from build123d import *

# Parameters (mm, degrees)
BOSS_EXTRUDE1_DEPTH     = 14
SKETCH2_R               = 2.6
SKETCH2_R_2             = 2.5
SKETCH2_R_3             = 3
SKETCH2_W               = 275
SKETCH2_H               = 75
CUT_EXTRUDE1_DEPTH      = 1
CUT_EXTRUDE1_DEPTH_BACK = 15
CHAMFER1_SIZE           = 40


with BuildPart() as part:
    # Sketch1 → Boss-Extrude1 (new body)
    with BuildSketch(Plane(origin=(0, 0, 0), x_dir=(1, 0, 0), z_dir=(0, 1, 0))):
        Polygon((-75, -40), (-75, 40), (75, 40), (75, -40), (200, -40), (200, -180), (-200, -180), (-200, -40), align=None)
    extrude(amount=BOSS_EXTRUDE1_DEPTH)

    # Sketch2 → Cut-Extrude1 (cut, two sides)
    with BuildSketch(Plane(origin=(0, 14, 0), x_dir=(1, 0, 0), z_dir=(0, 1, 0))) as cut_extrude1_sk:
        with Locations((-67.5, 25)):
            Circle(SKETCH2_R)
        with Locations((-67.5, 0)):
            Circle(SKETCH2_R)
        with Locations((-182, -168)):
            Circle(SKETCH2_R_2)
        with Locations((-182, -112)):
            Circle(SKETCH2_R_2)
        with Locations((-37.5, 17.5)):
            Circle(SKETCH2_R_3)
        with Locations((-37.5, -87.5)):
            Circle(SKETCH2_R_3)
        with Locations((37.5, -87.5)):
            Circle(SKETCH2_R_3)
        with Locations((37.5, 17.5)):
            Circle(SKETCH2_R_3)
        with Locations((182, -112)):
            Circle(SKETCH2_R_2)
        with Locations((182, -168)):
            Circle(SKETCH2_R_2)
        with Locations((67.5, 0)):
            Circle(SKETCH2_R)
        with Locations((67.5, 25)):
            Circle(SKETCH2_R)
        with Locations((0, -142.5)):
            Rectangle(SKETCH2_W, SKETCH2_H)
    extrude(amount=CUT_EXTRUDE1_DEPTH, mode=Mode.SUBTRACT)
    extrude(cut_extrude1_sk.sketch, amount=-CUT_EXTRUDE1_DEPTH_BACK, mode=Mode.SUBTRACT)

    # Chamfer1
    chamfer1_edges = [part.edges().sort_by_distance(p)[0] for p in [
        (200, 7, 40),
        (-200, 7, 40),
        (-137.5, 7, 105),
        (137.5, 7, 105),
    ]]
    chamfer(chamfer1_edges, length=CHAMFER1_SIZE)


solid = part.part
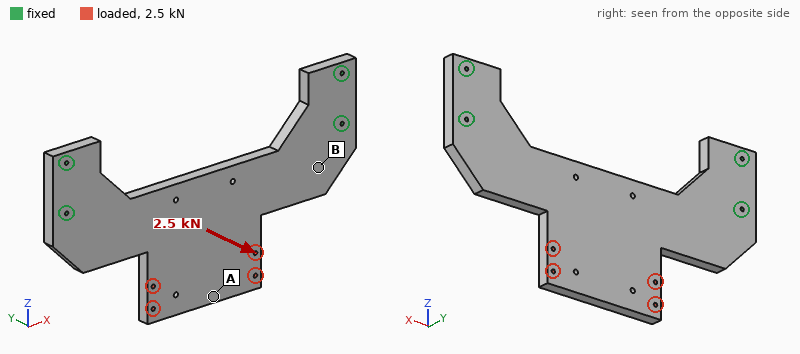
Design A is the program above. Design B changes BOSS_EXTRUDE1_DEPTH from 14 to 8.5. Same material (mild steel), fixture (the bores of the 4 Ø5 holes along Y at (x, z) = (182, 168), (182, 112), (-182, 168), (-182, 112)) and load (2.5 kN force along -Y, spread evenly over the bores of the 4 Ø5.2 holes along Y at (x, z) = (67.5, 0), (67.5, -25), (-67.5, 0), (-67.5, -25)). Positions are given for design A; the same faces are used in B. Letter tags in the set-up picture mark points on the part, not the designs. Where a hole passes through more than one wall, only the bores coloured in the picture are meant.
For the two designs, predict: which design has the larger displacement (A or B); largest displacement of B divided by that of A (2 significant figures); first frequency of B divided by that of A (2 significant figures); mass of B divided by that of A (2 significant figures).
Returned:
B
4.2
0.63
0.61
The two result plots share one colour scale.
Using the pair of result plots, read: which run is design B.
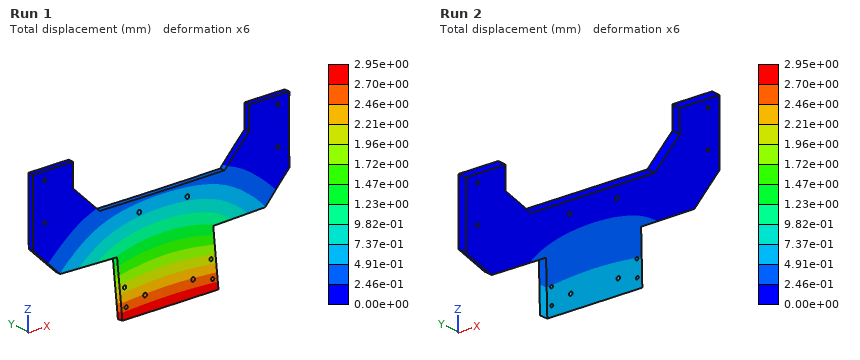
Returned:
Run 1
